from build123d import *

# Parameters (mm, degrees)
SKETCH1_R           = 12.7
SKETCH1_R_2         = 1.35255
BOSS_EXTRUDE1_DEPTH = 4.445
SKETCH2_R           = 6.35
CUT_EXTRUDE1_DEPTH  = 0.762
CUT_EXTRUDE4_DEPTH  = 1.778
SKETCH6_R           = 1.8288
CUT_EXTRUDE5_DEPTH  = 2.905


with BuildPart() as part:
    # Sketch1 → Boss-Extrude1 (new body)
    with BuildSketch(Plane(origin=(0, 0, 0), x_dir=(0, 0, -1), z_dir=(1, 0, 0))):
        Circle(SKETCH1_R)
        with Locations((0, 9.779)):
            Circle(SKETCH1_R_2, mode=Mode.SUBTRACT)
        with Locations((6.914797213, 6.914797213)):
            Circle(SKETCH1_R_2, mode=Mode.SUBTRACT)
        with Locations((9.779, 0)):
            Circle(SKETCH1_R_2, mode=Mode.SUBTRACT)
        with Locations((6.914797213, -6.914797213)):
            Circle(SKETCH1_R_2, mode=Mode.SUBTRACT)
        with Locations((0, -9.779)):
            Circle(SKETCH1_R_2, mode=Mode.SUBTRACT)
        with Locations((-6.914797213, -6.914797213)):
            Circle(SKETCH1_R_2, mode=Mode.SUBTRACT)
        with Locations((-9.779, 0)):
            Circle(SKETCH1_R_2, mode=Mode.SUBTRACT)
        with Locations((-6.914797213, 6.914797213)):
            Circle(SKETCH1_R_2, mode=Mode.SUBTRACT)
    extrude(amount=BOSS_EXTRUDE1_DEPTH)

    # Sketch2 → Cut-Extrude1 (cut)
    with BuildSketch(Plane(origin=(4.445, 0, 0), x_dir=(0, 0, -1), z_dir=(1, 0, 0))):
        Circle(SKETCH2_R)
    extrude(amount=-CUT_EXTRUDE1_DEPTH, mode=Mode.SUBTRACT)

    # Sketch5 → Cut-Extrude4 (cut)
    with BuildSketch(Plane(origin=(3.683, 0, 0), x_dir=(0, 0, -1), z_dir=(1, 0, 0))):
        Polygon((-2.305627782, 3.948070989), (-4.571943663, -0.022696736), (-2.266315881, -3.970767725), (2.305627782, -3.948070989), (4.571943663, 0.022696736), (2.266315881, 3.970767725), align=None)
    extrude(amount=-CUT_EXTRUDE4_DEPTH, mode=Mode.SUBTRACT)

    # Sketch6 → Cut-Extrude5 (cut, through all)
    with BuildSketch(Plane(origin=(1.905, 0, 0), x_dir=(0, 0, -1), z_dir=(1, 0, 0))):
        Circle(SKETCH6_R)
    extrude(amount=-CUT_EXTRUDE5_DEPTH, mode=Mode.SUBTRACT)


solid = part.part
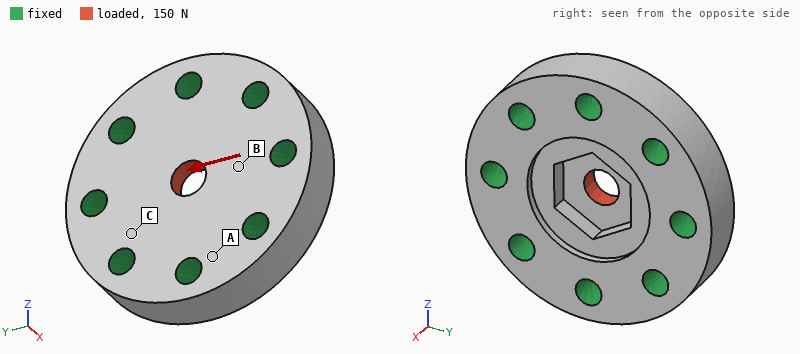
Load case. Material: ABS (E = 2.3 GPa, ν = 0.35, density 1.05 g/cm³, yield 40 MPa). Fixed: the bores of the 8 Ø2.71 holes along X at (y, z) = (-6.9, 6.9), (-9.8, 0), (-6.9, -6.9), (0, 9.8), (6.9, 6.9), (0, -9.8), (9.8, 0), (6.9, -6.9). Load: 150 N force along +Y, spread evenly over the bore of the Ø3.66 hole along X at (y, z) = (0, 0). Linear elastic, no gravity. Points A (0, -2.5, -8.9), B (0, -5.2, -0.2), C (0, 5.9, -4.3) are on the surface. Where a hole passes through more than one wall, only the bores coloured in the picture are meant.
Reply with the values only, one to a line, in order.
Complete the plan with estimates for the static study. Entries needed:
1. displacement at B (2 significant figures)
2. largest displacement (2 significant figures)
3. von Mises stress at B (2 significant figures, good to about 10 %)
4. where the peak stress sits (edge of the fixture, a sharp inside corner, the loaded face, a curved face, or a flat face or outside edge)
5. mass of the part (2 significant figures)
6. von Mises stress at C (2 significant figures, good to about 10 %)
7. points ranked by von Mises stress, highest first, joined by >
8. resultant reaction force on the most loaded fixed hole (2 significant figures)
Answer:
5.5 µm
13 µm
3.8 MPa
the loaded face
1.9 g
2.1 MPa
B > C > A
34 N
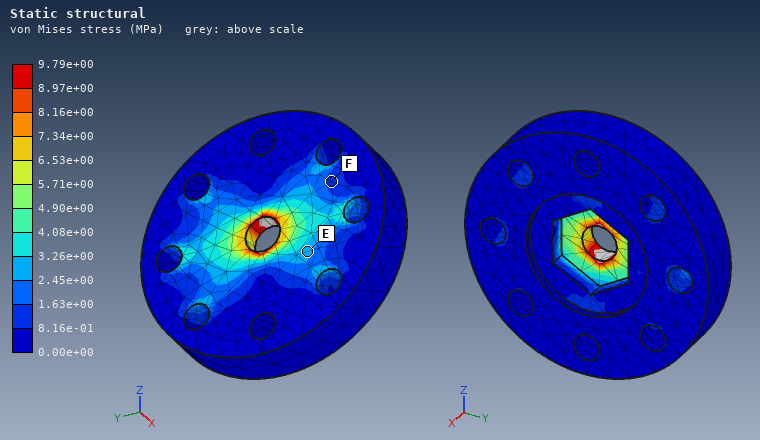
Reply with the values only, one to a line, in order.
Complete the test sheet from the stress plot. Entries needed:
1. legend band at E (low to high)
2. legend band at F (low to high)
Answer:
2.45e+00 to 3.26e+00 MPa
8.16e-01 to 1.63e+00 MPa
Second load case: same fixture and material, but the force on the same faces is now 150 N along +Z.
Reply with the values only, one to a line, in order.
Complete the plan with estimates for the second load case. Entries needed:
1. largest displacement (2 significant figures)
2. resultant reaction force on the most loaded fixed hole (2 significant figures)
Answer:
13 µm
34 N
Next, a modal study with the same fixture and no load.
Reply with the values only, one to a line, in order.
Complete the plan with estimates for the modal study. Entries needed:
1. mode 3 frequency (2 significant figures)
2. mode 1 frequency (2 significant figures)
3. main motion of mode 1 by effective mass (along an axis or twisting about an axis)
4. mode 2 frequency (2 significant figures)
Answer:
38 kHz
29 kHz
along X
38 kHz
